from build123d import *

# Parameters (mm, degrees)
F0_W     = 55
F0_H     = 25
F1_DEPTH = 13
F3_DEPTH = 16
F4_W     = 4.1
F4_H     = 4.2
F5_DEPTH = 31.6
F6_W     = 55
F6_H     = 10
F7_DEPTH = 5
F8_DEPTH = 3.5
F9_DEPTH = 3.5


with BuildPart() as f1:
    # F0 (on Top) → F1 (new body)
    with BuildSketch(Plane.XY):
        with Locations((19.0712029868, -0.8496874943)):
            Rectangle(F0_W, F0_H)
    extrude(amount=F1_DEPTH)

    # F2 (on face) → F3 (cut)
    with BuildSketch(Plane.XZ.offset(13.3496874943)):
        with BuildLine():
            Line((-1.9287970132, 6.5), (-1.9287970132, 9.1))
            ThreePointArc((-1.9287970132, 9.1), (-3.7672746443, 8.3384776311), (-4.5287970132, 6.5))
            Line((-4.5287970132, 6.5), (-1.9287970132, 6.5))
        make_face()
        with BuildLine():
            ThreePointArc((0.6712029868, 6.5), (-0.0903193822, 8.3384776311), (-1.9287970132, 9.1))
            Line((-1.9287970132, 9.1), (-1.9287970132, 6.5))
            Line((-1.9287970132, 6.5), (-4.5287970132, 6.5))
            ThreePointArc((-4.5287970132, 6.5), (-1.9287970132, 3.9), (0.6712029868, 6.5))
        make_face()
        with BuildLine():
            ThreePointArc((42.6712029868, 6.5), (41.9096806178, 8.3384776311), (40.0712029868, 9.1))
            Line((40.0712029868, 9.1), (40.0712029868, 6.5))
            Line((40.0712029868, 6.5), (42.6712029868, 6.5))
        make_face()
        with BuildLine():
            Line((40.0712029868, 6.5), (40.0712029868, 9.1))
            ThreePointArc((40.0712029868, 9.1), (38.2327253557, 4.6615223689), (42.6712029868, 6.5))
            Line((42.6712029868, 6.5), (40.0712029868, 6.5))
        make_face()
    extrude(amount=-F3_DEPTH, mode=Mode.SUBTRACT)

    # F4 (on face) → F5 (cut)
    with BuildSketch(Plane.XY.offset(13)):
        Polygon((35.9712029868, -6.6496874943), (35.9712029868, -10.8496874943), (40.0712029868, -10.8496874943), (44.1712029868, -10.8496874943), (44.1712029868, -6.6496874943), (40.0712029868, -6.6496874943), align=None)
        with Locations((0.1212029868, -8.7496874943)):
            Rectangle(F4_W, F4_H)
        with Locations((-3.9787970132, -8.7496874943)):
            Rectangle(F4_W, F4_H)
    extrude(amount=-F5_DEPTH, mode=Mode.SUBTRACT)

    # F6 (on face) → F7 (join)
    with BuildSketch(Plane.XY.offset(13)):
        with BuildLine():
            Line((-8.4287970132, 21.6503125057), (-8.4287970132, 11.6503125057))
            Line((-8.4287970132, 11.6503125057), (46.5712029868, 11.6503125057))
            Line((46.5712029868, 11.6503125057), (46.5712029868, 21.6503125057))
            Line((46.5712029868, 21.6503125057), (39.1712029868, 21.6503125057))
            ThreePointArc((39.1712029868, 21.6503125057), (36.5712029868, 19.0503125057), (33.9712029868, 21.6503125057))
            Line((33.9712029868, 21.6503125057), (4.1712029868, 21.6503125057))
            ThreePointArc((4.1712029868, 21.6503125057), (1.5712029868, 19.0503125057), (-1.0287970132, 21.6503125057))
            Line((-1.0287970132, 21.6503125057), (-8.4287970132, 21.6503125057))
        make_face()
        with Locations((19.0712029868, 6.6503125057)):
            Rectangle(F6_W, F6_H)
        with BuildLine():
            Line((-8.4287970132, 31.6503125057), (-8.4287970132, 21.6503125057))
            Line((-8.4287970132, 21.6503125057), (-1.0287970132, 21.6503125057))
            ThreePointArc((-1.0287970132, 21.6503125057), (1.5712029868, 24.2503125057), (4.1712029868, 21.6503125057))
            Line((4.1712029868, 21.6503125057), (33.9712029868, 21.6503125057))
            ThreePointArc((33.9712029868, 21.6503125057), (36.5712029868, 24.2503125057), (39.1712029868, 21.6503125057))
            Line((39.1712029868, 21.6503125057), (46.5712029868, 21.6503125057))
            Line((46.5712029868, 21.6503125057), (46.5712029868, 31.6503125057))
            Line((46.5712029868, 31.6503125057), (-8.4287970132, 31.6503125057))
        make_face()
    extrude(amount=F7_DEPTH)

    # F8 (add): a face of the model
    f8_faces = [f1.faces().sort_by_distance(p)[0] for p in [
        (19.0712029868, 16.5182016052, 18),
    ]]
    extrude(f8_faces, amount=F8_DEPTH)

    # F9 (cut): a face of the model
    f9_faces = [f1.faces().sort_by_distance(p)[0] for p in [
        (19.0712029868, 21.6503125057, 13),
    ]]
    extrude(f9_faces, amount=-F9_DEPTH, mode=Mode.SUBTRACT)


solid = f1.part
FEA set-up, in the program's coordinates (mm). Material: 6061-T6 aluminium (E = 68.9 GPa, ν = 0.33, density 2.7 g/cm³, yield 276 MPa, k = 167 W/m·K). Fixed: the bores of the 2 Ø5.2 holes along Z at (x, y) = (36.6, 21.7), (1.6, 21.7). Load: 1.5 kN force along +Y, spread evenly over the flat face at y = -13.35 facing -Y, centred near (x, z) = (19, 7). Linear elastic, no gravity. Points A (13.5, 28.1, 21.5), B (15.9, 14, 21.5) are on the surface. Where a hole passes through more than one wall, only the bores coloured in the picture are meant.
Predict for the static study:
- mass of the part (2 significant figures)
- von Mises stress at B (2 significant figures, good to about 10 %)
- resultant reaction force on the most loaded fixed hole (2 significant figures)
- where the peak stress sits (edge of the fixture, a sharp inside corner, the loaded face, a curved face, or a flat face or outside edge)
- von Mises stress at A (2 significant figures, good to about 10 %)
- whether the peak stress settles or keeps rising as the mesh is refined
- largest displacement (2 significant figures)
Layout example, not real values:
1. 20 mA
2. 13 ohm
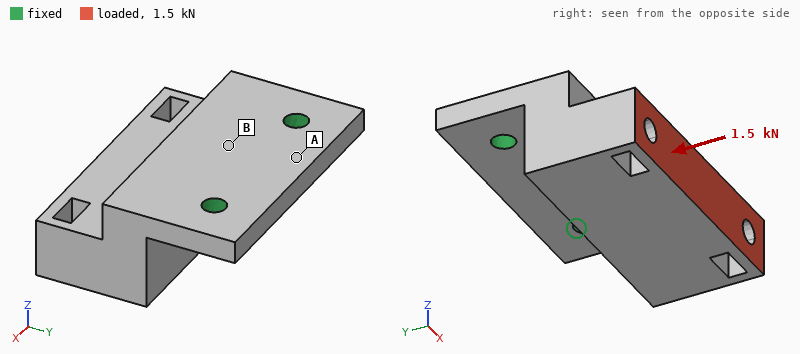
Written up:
1. 71 g
2. 58 MPa
3. 760 N
4. edge of the fixture
5. 16 MPa
6. keeps rising
7. 0.21 mm
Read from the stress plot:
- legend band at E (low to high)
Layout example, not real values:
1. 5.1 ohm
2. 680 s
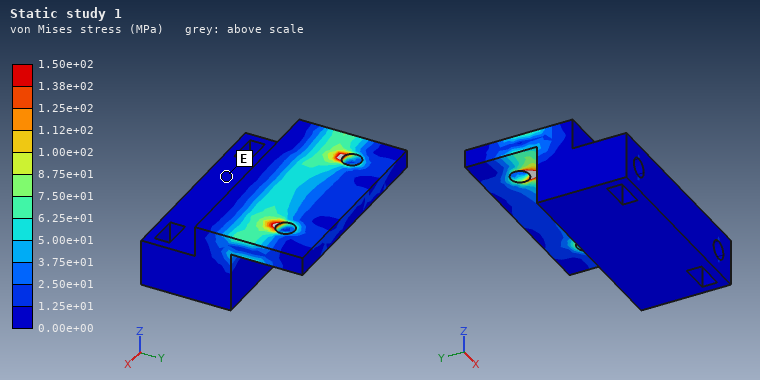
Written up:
1. 0.00e+00 to 1.25e+01 MPa
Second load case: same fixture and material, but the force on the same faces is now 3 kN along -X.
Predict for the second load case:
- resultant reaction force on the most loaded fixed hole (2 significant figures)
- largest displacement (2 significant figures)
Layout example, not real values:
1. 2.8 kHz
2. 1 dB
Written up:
1. 3.3 kN
2. 46 µm
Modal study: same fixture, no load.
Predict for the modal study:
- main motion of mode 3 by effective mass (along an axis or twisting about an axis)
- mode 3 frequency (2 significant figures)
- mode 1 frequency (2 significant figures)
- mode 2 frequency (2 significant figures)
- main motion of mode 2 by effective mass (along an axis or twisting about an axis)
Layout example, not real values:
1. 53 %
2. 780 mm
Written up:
1. along X
2. 9200 Hz
3. 1800 Hz
4. 6200 Hz
5. along X
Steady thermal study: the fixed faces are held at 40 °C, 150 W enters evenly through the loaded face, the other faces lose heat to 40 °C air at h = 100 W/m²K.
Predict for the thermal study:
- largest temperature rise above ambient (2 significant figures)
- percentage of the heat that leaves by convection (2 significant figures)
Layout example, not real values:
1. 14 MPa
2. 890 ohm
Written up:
1. 82 K
2. 23 %
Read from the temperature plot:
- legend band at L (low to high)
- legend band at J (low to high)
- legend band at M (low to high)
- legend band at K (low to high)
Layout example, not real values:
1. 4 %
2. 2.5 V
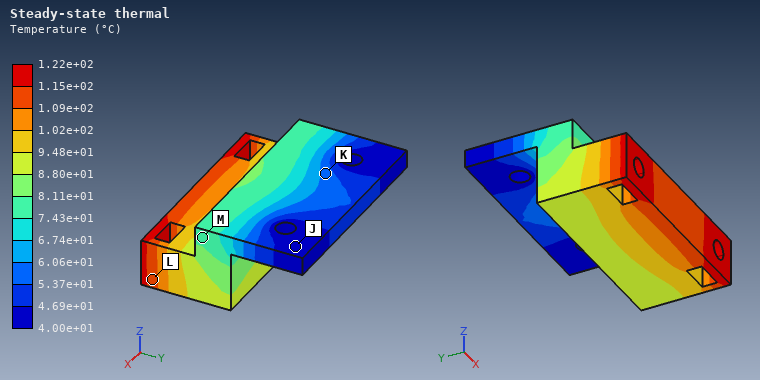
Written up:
1. 1.09e+02 to 1.15e+02 °C
2. 4.00e+01 to 4.69e+01 °C
3. 7.43e+01 to 8.11e+01 °C
4. 5.37e+01 to 6.06e+01 °C
